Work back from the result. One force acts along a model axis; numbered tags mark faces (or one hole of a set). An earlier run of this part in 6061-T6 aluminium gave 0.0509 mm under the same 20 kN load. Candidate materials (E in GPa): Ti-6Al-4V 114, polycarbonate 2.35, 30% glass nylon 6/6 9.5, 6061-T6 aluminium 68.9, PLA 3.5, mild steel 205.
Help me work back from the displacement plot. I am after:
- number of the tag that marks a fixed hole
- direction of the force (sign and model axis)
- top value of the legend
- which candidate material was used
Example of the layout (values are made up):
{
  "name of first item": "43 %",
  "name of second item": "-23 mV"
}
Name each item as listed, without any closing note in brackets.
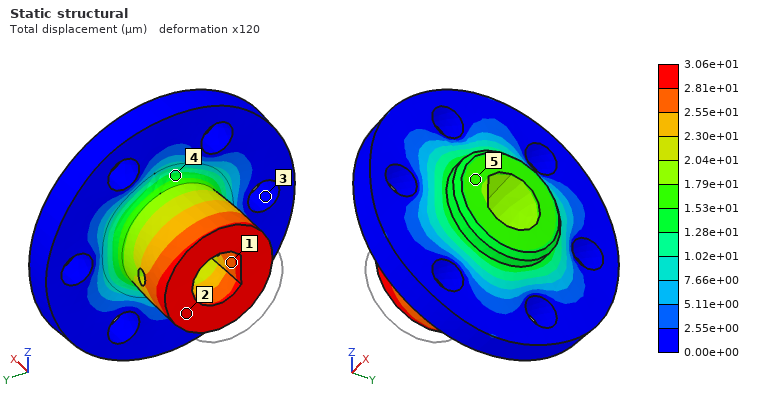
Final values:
{
  "number of the tag that marks a fixed hole": "3",
  "direction of the force": "+X",
  "top value of the legend": "3.06e+01 µm",
  "which candidate material was used": "Ti-6Al-4V"
}
